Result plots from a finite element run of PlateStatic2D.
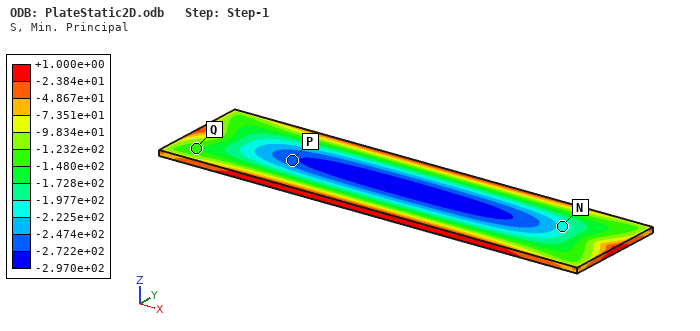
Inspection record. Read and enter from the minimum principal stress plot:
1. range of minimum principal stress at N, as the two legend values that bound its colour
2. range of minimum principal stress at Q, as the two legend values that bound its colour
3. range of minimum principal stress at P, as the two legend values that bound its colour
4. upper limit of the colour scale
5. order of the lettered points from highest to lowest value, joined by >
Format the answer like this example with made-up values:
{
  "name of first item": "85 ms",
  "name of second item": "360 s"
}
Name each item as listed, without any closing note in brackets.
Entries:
{
  "range of minimum principal stress at N, as the two legend values that bound its colour": "-2.225e+02 to -1.977e+02",
  "range of minimum principal stress at Q, as the two legend values that bound its colour": "-1.480e+02 to -1.232e+02",
  "range of minimum principal stress at P, as the two legend values that bound its colour": "-2.722e+02 to -2.474e+02",
  "upper limit of the colour scale": "+1.000e+00",
  "order of the lettered points from highest to lowest value, joined by >": "Q > N > P"
}
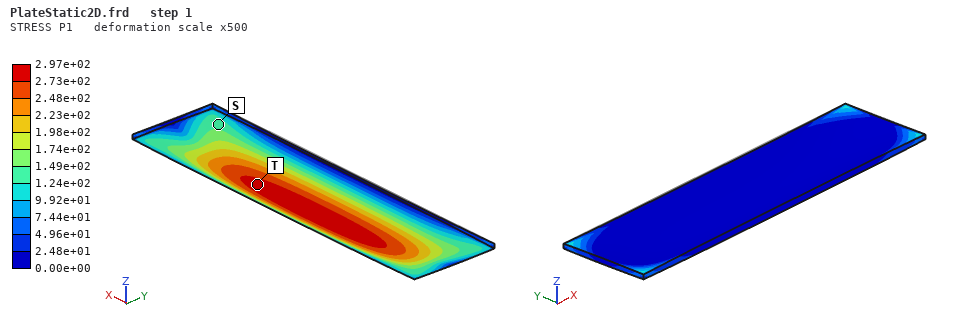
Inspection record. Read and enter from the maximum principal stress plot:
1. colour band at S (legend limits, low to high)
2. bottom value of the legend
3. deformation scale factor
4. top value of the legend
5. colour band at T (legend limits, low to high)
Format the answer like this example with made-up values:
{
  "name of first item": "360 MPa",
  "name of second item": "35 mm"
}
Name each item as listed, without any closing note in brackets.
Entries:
{
  "colour band at S": "1.24e+02 to 1.49e+02",
  "bottom value of the legend": "0.00e+00",
  "deformation scale factor": "500",
  "top value of the legend": "2.97e+02",
  "colour band at T": "2.73e+02 to 2.97e+02"
}
